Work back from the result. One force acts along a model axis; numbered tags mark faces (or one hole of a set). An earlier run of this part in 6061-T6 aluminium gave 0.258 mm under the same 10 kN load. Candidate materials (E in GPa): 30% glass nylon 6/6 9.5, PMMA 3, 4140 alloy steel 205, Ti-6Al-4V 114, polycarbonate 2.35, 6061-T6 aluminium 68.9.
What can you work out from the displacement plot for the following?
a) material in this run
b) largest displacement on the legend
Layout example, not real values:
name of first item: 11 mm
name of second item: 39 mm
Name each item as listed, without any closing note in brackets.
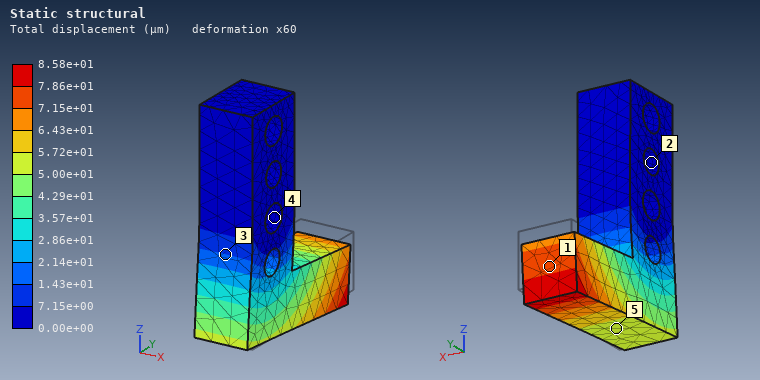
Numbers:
material in this run: 4140 alloy steel
largest displacement on the legend: 8.58e+01 µm
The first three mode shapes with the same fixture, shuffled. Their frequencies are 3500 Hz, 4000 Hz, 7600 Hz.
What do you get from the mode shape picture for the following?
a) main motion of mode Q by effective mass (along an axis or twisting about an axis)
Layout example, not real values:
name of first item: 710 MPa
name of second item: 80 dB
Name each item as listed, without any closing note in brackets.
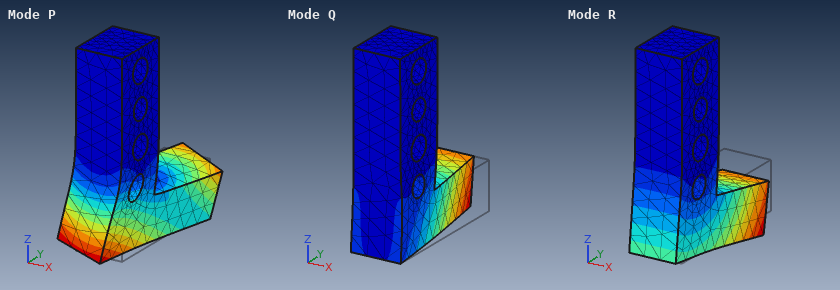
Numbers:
main motion of mode Q by effective mass: along X
